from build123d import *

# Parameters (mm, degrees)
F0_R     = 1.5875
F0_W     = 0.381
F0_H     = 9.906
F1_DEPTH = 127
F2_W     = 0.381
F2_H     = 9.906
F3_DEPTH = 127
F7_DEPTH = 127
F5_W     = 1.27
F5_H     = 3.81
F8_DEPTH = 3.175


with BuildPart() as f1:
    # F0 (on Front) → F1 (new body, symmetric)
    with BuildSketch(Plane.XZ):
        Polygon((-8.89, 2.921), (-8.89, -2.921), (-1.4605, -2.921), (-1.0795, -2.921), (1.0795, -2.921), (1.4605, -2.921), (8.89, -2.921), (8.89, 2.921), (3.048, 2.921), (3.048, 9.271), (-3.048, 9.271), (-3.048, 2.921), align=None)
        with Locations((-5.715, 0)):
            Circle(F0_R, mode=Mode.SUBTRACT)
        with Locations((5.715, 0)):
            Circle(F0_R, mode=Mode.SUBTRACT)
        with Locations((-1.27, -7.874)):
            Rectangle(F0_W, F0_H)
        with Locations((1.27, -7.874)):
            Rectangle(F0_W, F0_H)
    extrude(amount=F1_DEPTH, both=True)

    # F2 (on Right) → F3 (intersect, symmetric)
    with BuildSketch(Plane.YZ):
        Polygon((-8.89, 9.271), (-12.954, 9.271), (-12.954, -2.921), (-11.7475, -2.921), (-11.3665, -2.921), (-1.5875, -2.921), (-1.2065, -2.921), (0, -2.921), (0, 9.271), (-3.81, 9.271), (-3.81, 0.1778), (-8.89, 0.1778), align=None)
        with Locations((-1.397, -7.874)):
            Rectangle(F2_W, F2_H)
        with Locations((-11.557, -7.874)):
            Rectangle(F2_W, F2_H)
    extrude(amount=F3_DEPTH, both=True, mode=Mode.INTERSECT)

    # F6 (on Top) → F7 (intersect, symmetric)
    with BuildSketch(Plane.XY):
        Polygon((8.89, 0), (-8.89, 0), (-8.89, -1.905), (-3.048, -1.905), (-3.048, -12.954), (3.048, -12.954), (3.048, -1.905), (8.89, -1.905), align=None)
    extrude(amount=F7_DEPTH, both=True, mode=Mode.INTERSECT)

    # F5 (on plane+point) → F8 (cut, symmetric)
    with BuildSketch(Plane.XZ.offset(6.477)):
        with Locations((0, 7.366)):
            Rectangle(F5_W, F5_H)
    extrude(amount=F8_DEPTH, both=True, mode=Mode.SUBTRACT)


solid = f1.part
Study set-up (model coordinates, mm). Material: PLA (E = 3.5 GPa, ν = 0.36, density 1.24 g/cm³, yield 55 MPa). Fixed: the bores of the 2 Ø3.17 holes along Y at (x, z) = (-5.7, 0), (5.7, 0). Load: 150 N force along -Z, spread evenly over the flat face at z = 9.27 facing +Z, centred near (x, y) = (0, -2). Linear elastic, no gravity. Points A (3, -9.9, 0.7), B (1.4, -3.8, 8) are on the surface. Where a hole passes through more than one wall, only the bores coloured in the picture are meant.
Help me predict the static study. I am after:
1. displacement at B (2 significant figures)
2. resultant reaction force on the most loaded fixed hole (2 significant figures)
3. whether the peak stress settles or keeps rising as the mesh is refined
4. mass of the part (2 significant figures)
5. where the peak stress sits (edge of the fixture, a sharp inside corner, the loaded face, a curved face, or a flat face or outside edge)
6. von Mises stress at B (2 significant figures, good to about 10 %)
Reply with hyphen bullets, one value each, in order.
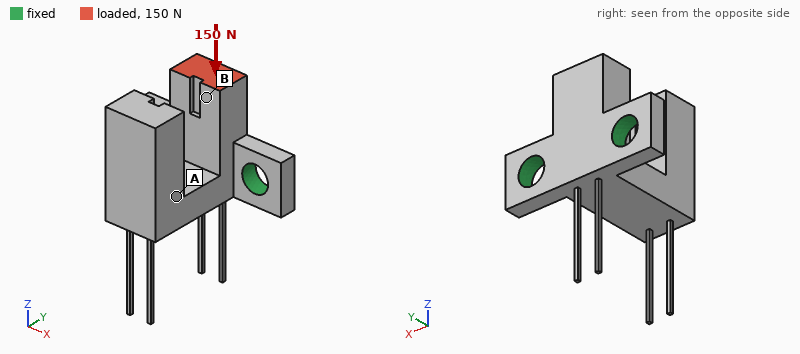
- 0.080 mm
- 77 N
- keeps rising
- 0.97 g
- edge of the fixture
- 6.7 MPa
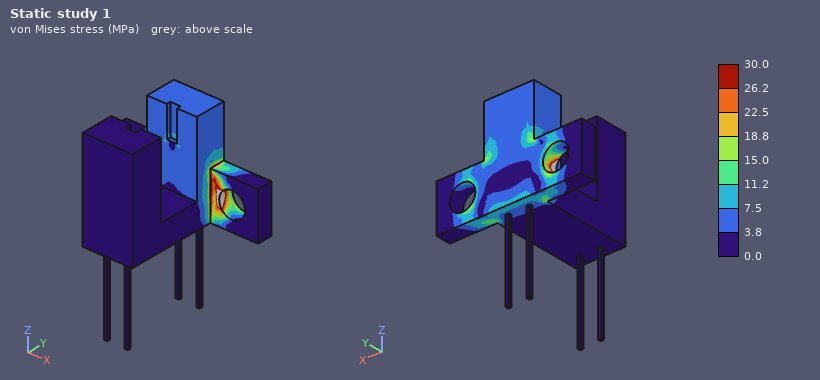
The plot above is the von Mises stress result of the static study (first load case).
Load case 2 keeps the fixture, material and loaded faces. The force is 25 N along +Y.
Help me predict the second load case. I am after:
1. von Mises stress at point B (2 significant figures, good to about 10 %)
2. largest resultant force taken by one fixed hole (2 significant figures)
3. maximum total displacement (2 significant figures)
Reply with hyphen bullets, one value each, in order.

- 2.7 MPa
- 17 N
- 0.17 mm
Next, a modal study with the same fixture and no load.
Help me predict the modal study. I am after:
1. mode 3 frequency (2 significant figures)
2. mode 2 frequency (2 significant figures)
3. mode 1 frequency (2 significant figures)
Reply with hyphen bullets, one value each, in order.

- 1000 Hz
- 1000 Hz
- 1000 Hz
